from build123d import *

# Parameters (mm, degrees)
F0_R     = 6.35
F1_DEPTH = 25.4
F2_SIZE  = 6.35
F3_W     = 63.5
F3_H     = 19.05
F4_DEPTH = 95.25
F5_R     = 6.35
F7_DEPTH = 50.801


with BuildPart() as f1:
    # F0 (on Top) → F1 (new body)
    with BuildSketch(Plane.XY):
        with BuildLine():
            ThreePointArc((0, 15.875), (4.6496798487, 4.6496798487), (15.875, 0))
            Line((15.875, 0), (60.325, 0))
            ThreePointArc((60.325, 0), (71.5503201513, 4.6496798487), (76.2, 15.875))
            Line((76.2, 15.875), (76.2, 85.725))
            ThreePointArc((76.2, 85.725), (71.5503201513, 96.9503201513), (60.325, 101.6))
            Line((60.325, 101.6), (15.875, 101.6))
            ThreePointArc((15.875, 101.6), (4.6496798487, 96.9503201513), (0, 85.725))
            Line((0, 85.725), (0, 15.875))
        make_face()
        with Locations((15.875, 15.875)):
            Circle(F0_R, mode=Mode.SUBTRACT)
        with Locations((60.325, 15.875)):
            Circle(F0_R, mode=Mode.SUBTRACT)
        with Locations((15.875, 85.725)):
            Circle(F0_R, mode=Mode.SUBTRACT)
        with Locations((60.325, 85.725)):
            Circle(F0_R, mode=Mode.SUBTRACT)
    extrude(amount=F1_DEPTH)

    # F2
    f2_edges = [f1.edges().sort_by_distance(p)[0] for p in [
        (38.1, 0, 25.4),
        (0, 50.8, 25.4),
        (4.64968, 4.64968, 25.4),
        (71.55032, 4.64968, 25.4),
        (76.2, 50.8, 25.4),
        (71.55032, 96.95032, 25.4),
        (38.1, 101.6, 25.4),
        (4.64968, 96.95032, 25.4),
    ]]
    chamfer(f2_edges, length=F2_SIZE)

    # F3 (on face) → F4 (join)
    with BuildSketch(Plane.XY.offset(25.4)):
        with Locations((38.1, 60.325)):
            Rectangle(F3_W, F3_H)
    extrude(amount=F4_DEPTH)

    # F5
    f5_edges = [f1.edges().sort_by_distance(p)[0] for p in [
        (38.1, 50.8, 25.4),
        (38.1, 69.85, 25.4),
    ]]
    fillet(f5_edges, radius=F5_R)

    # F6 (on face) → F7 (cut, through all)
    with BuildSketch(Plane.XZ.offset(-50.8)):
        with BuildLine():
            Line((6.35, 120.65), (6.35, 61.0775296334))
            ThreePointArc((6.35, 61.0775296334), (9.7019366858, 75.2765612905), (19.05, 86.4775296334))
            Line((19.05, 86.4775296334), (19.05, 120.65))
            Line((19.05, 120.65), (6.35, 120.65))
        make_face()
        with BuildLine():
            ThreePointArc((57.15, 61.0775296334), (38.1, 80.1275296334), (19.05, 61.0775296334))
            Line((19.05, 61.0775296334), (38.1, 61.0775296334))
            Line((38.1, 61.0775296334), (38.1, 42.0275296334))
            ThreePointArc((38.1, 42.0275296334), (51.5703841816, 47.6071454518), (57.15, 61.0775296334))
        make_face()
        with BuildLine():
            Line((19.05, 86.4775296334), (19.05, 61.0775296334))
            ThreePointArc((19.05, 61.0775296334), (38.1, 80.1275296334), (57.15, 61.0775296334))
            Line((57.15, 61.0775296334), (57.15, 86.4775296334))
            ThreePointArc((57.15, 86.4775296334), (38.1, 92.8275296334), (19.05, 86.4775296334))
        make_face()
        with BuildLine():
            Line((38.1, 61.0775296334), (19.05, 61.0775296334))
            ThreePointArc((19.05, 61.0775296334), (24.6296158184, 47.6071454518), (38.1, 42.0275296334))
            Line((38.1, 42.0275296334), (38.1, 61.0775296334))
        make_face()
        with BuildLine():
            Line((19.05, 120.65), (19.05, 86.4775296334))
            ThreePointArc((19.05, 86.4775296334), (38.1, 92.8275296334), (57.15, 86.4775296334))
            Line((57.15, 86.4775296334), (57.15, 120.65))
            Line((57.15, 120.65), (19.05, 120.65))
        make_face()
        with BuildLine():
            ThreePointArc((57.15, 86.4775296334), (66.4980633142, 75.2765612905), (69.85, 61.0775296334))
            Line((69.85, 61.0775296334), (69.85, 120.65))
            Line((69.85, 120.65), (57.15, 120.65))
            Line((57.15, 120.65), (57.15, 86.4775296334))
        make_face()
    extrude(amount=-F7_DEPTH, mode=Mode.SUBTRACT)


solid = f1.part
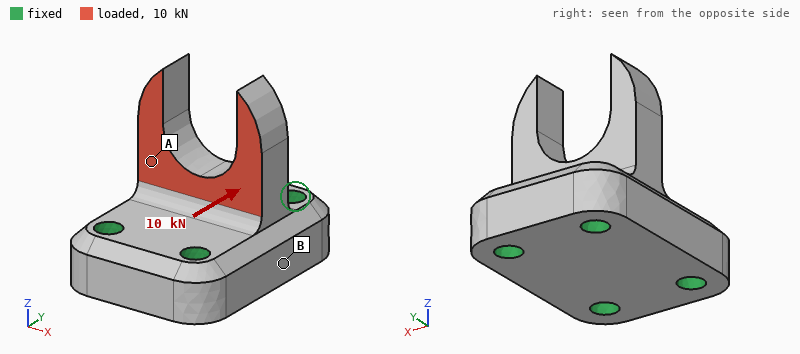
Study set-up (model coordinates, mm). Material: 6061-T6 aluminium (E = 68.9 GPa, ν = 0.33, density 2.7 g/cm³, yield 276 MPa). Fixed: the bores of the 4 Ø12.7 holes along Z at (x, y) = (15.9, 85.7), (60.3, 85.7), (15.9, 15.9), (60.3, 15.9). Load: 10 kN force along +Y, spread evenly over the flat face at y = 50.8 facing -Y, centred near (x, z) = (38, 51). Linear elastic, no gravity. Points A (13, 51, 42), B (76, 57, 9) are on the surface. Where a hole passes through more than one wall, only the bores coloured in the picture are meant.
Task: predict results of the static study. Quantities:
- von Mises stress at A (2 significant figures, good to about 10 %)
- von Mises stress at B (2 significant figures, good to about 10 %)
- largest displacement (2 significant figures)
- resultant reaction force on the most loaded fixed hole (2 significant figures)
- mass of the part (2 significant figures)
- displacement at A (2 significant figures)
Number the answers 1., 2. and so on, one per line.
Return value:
1. 45 MPa
2. 9.2 MPa
3. 0.15 mm
4. 4.5 kN
5. 580 g
6. 0.034 mm
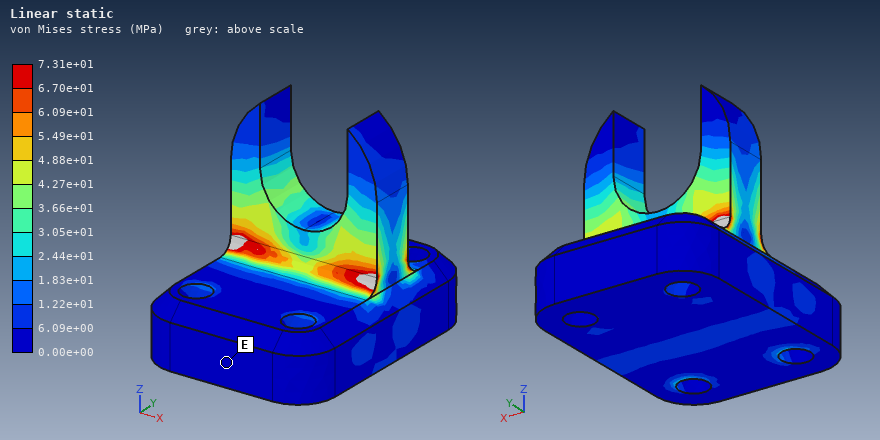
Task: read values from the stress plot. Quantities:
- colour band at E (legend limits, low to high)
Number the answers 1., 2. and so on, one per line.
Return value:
1. 0.00e+00 to 6.09e+00 MPa
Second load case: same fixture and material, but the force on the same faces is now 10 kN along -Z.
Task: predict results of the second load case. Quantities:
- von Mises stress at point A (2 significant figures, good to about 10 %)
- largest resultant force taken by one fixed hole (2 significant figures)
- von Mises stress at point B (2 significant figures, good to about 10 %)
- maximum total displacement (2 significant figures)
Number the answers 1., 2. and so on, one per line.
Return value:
1. 36 MPa
2. 2.6 kN
3. 4.9 MPa
4. 81 µm
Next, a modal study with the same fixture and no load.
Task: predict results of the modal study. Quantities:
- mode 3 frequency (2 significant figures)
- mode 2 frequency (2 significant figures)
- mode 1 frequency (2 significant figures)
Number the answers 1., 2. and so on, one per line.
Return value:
1. 6600 Hz
2. 6100 Hz
3. 5900 Hz
